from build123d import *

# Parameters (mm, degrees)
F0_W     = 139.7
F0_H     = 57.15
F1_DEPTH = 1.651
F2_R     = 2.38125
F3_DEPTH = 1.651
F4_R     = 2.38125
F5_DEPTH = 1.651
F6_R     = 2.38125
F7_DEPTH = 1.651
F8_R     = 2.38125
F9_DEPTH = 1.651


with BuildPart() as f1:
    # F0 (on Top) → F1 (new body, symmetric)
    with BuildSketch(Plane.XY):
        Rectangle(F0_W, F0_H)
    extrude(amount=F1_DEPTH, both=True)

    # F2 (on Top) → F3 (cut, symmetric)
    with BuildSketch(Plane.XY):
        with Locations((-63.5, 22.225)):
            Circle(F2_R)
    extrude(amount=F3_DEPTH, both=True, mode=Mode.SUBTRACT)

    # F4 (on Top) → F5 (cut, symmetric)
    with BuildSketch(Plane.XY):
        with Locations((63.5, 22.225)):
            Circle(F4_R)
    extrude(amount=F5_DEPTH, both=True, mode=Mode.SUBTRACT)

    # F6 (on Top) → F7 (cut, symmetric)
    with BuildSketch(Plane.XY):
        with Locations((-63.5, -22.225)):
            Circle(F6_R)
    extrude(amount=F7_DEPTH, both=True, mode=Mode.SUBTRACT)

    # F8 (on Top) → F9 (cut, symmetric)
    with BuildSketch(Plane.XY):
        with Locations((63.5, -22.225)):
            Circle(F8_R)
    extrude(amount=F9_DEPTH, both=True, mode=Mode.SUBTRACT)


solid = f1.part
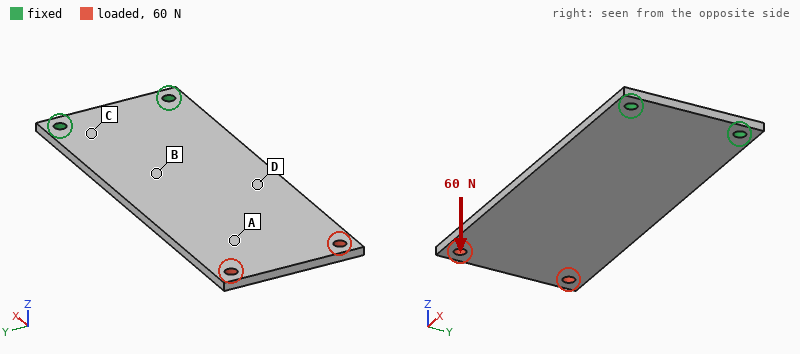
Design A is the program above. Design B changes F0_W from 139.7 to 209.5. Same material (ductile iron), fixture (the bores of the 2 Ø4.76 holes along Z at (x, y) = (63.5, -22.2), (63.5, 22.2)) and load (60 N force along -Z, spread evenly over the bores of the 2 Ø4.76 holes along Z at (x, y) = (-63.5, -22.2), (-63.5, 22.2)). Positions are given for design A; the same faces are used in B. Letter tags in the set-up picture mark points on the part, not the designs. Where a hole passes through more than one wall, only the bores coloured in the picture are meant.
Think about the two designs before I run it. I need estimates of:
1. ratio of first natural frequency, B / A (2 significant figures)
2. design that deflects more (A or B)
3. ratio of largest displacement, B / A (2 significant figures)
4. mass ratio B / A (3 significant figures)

0.64
B
1.3
1.50
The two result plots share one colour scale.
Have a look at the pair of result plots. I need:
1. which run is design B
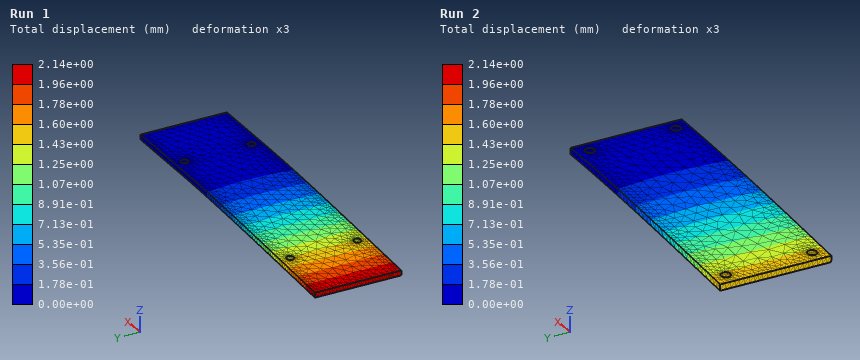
Run 1
